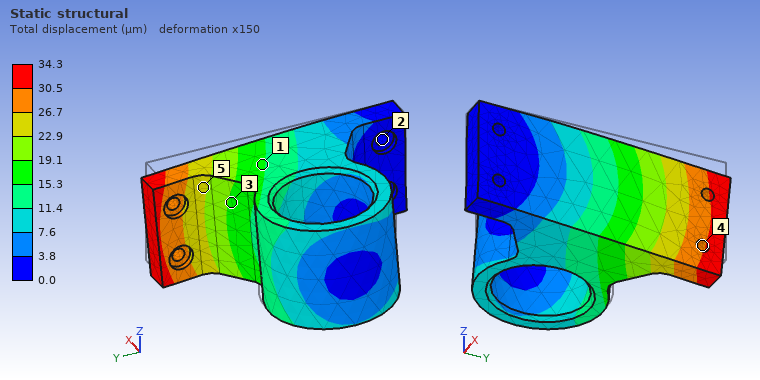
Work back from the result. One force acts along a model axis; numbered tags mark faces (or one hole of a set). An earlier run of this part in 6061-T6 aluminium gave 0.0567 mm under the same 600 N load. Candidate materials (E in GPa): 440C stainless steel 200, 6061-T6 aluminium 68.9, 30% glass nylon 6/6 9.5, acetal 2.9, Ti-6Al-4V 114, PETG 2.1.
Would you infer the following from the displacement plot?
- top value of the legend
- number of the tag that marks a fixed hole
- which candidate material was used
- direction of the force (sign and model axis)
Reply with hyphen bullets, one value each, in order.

- 34.3 µm
- 2
- Ti-6Al-4V
- -Z
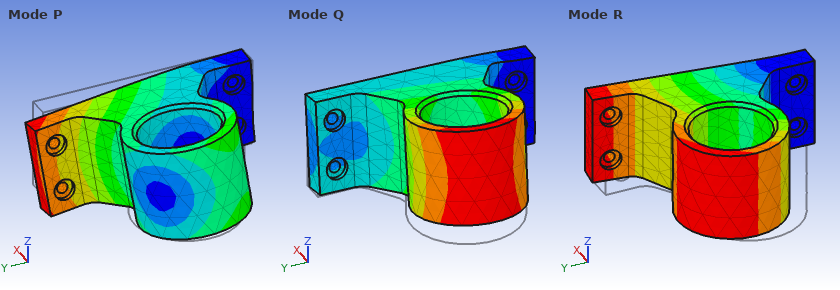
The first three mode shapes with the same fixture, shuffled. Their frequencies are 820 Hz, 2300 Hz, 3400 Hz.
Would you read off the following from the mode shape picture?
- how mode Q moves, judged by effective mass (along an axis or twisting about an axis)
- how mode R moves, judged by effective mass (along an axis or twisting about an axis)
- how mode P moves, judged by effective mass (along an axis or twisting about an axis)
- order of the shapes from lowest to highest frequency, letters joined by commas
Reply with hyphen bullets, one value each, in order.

- along Z
- along X
- along Z
- R, Q, P
